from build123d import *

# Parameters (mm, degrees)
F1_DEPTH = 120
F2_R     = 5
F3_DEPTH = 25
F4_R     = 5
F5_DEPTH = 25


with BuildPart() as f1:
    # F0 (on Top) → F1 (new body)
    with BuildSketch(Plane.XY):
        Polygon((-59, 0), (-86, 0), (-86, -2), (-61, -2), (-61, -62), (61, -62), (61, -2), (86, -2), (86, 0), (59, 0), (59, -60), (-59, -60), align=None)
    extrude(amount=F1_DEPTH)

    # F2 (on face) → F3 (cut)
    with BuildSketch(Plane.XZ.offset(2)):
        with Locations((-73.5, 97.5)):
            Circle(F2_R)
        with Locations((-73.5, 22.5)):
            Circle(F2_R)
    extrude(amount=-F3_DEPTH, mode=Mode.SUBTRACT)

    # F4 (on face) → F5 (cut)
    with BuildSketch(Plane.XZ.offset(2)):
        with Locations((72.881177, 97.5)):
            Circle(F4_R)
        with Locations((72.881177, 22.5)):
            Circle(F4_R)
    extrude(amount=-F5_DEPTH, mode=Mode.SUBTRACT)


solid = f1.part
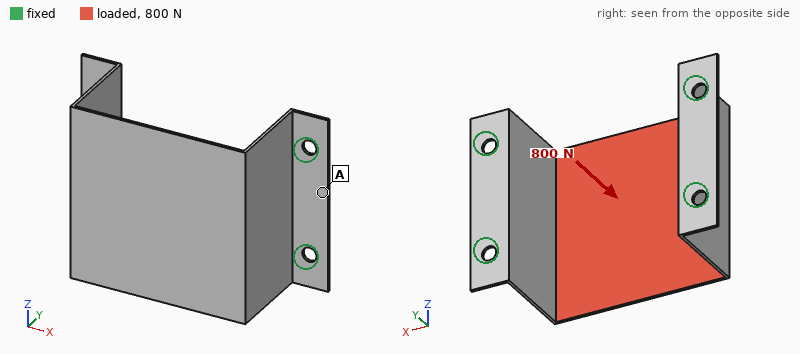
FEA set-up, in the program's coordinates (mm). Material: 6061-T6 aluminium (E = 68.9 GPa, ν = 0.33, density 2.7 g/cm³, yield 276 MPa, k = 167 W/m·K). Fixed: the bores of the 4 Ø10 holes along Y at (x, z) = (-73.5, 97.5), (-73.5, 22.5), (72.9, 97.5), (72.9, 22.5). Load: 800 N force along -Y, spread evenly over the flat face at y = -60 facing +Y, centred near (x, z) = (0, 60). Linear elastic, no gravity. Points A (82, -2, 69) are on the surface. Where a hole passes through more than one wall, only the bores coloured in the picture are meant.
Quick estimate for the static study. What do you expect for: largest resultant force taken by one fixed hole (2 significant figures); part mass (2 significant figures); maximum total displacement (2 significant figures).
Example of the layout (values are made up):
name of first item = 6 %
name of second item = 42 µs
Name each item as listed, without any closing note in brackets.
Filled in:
largest resultant force taken by one fixed hole = 220 N
part mass = 190 g
maximum total displacement = 1.2 mm
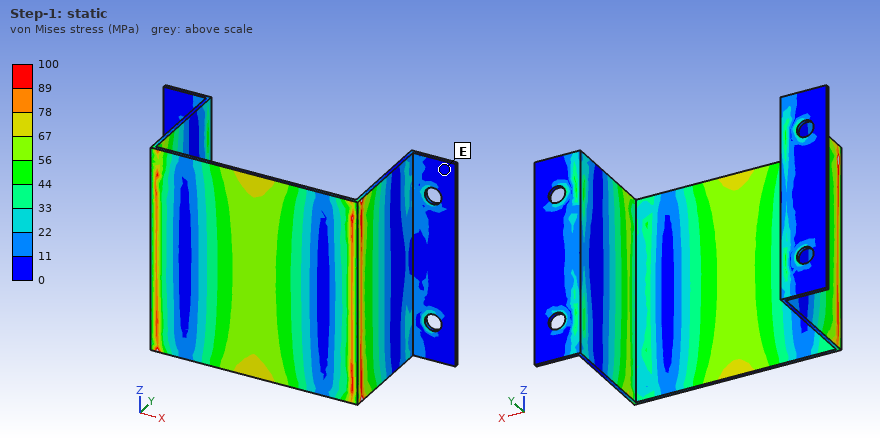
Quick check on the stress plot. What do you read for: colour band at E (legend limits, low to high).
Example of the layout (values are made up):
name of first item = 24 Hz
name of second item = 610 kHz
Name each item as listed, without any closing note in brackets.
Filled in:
colour band at E = 0 to 11 MPa
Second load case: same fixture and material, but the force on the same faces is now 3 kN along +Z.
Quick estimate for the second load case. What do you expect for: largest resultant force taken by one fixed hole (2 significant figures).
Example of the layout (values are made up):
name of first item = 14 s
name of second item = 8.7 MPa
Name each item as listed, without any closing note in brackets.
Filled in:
largest resultant force taken by one fixed hole = 1.4 kN
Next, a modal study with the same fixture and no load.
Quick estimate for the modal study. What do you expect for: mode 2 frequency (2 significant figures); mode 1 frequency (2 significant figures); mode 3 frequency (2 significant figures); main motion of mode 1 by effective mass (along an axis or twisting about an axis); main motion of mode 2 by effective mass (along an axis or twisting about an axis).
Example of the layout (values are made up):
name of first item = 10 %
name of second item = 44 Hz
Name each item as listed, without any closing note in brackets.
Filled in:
mode 2 frequency = 550 Hz
mode 1 frequency = 260 Hz
mode 3 frequency = 720 Hz
main motion of mode 1 by effective mass = along X
main motion of mode 2 by effective mass = along Y
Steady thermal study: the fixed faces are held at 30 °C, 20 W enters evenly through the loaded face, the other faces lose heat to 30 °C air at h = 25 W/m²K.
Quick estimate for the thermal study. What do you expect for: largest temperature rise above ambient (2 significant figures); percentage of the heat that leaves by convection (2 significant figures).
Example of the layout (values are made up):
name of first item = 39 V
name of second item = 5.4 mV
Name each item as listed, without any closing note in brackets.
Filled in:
largest temperature rise above ambient = 16 K
percentage of the heat that leaves by convection = 53 %
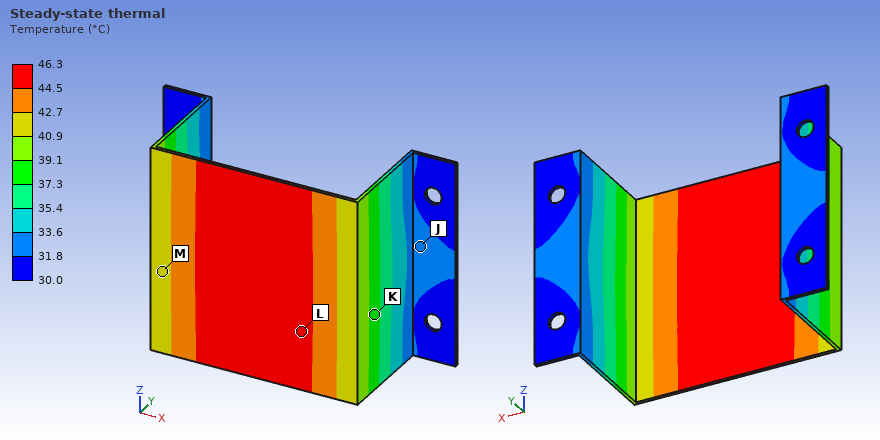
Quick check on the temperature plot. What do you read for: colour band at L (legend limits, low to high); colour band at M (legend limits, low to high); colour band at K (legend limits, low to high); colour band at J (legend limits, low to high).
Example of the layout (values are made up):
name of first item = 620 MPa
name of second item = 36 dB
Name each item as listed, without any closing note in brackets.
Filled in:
colour band at L = 44.5 to 46.3 °C
colour band at M = 40.9 to 42.7 °C
colour band at K = 37.3 to 39.1 °C
colour band at J = 31.8 to 33.6 °C
